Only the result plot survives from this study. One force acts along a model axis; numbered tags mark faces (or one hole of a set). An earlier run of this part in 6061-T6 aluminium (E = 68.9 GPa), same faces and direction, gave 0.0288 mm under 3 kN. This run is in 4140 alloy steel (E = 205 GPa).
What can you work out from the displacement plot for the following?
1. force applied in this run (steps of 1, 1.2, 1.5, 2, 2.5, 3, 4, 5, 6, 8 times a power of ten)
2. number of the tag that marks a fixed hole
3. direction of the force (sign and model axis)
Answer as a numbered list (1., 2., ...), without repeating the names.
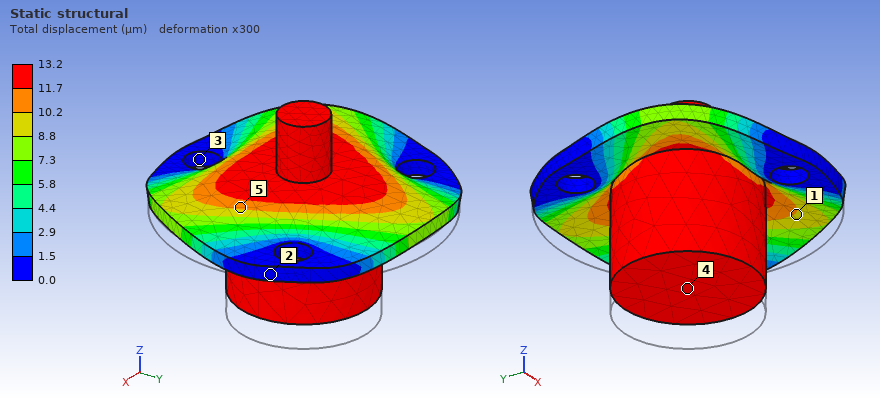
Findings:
1. 4 kN
2. 3
3. +Z
